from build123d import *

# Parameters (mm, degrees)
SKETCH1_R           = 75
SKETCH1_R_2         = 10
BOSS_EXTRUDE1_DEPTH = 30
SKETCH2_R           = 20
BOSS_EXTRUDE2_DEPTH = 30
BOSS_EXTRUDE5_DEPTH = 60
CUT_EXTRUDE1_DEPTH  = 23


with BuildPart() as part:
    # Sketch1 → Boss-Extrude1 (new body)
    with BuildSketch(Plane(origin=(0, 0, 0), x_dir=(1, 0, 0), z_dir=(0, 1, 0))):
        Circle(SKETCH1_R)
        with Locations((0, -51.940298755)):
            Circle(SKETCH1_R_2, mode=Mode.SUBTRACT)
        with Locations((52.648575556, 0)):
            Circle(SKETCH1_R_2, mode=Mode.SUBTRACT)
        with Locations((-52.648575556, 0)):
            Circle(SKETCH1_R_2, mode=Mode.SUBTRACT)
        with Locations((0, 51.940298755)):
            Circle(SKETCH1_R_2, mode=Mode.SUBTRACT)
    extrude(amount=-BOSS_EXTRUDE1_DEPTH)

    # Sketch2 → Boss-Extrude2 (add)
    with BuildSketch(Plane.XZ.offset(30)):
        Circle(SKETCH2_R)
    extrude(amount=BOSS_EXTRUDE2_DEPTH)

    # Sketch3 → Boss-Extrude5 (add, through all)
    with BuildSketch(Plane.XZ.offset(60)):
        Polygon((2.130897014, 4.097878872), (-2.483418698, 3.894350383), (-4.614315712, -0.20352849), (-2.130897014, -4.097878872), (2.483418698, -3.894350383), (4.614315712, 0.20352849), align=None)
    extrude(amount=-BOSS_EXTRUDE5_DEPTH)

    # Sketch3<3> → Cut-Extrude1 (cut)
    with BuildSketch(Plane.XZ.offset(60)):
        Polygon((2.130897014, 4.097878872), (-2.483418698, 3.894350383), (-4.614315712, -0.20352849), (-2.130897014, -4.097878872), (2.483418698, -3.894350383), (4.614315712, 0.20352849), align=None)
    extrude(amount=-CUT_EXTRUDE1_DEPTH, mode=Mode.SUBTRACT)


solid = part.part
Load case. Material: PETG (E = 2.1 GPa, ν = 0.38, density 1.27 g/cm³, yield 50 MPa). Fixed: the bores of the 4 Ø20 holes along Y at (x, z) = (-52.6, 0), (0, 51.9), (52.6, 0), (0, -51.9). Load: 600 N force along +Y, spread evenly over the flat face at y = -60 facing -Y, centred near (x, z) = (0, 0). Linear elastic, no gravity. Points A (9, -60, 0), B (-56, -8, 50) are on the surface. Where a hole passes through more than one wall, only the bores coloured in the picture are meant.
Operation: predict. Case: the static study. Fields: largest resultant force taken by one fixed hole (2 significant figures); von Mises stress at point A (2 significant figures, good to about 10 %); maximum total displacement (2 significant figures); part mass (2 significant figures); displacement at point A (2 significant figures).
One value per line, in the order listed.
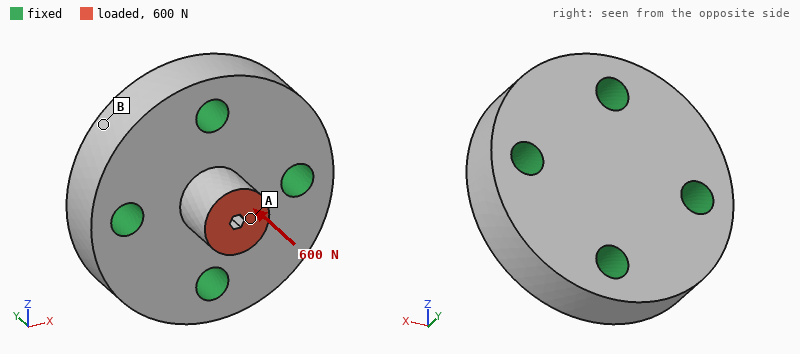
160 N
0.52 MPa
15 µm
670 g
15 µm
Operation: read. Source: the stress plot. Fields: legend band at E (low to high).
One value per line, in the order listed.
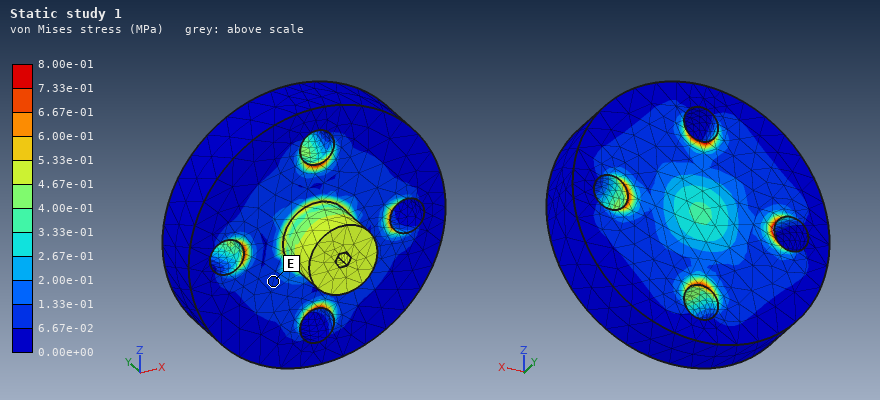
6.67e-02 to 1.33e-01 MPa
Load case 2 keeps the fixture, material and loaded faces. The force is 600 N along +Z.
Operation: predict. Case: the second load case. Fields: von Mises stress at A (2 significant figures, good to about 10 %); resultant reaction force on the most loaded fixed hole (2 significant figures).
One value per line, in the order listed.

0.98 MPa
360 N
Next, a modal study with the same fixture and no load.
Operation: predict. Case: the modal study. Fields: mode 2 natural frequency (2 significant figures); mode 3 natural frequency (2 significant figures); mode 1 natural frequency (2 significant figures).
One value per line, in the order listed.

3100 Hz
3500 Hz
3100 Hz
